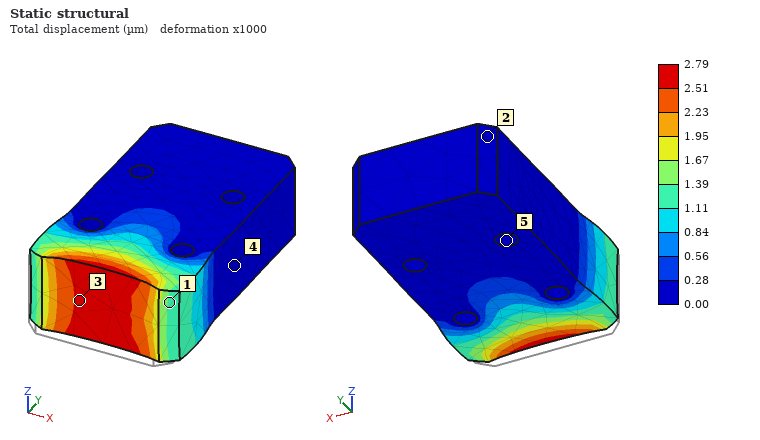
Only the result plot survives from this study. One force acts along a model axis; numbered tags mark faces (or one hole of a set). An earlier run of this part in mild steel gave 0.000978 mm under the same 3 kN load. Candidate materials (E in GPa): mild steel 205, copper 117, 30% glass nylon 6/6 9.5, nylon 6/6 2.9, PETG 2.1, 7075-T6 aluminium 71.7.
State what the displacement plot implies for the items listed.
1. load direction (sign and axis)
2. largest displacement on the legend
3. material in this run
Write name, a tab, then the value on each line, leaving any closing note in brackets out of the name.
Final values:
load direction	+Y
largest displacement on the legend	2.79 µm
material in this run	7075-T6 aluminium
